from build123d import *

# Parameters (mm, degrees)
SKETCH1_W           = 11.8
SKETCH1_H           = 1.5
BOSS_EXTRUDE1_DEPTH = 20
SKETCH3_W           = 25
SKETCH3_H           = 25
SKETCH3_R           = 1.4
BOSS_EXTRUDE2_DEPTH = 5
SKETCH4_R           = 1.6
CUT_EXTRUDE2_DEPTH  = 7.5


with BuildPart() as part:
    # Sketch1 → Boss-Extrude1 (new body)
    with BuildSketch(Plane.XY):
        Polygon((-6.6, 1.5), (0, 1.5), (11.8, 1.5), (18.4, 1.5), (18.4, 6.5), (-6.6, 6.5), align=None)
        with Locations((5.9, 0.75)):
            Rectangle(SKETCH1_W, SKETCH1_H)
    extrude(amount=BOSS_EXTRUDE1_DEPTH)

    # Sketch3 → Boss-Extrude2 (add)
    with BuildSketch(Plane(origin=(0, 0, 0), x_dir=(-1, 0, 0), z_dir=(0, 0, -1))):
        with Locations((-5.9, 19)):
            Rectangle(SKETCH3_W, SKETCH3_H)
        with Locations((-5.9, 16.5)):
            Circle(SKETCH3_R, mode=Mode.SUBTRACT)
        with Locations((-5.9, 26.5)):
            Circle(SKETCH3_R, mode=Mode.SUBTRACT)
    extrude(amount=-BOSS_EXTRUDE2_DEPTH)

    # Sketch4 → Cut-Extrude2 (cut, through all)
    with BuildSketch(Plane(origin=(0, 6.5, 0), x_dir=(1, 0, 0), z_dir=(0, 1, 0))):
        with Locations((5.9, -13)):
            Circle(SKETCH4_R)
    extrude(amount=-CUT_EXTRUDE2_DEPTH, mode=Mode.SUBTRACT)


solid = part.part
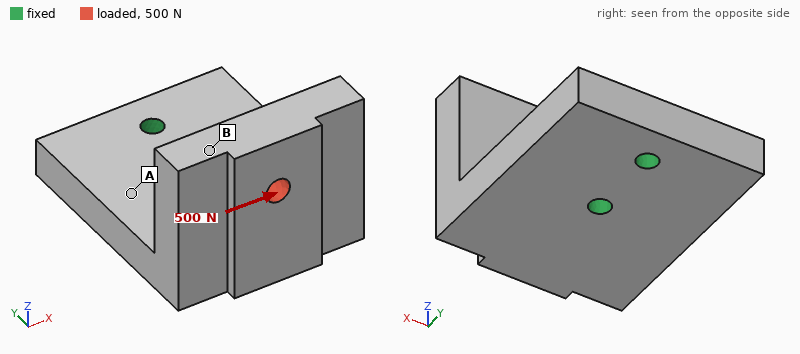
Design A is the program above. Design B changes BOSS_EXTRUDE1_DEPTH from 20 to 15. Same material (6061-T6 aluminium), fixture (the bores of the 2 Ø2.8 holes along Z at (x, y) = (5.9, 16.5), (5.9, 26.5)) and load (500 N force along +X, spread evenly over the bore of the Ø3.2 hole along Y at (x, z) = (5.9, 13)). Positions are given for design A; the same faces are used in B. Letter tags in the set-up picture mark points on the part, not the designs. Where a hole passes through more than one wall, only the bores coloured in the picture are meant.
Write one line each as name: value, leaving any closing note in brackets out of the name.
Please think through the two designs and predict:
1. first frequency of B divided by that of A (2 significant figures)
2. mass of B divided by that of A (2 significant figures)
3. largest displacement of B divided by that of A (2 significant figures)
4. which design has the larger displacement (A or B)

first frequency of B divided by that of A: 1.4
mass of B divided by that of A: 0.88
largest displacement of B divided by that of A: 0.84
which design has the larger displacement: A
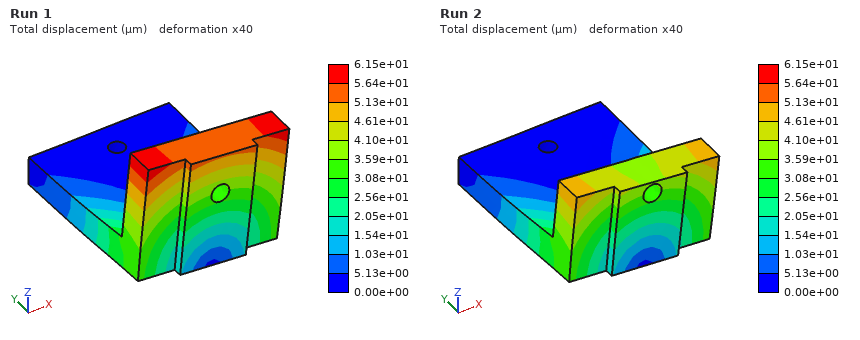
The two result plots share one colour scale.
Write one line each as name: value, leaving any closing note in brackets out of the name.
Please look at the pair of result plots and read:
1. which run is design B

which run is design B: Run 2
